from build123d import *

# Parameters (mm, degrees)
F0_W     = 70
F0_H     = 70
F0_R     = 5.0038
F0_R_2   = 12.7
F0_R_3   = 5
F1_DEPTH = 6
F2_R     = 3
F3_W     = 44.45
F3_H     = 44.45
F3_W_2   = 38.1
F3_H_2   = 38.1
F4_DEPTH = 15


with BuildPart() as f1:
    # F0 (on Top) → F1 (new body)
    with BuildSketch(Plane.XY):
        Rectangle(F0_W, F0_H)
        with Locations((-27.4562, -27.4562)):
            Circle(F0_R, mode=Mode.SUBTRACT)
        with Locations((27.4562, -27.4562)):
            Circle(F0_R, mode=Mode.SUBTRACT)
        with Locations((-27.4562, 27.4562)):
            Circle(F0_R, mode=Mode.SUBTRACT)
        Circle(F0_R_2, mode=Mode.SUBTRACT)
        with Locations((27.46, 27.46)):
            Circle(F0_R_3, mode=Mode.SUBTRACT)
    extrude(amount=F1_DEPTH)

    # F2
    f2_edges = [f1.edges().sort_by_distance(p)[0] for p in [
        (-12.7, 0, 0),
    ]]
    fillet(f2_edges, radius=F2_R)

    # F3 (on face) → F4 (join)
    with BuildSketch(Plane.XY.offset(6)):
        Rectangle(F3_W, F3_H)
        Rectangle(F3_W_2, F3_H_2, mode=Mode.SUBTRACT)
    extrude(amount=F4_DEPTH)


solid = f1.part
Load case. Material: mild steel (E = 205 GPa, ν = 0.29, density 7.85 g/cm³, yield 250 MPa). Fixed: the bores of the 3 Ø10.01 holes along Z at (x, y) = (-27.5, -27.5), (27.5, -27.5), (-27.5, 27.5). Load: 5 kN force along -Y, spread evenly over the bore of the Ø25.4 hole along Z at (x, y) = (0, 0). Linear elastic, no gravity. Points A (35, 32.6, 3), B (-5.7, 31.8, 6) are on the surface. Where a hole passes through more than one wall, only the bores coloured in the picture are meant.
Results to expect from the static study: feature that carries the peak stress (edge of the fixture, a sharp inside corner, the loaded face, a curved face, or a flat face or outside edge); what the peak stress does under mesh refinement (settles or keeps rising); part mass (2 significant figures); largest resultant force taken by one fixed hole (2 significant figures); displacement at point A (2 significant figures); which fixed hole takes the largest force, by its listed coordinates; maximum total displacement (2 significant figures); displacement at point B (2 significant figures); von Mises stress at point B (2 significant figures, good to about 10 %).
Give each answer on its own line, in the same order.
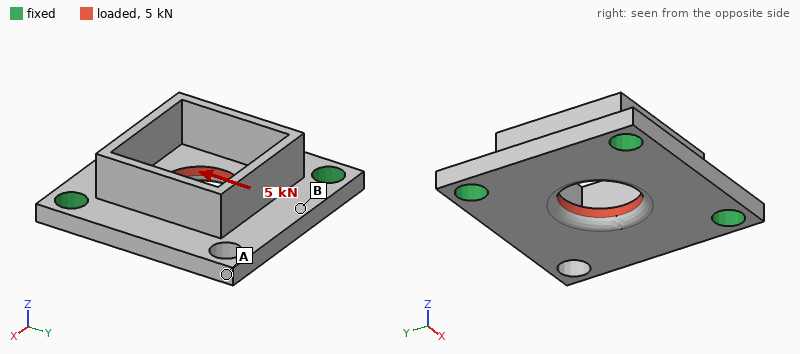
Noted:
edge of the fixture
keeps rising
250 g
2.2 kN
5.4 µm
(27.5, -27.5)
5.6 µm
2.7 µm
7.1 MPa
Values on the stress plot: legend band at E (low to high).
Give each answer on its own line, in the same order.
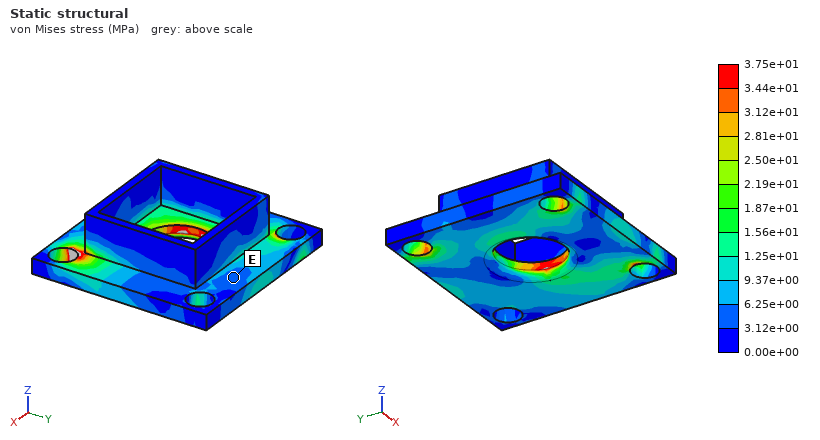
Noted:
3.12e+00 to 6.25e+00 MPa
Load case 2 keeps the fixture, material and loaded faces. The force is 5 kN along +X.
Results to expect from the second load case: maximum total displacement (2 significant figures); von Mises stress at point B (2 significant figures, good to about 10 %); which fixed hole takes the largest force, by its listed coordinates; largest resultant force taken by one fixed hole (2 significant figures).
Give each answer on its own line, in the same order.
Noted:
5.6 µm
8.8 MPa
(-27.5, 27.5)
2.2 kN
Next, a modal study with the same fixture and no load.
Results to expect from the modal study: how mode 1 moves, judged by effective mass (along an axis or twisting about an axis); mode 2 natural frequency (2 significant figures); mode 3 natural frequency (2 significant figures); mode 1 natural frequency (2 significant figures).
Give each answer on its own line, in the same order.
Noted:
along Z
12 kHz
12 kHz
2900 Hz
